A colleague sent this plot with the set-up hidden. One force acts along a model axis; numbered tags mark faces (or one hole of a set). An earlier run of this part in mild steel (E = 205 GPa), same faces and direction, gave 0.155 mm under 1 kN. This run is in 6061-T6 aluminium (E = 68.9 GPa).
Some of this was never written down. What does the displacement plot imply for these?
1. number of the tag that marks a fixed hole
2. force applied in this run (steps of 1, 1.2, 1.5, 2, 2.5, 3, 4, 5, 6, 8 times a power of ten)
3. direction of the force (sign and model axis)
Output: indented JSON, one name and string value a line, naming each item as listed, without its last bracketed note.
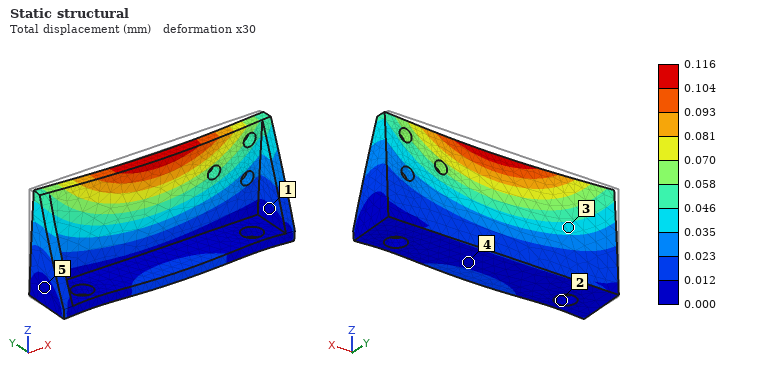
{
  "number of the tag that marks a fixed hole": "2",
  "force applied in this run": "250 N",
  "direction of the force": "-Y"
}
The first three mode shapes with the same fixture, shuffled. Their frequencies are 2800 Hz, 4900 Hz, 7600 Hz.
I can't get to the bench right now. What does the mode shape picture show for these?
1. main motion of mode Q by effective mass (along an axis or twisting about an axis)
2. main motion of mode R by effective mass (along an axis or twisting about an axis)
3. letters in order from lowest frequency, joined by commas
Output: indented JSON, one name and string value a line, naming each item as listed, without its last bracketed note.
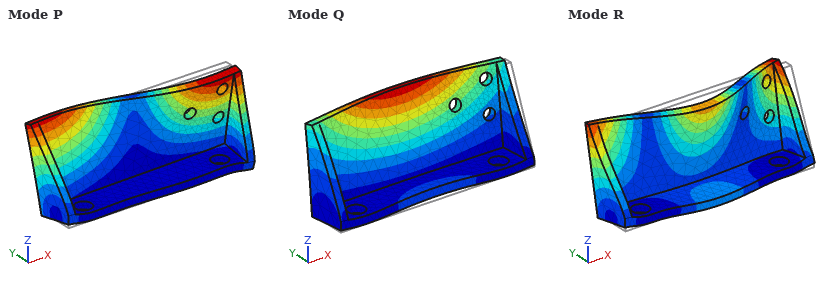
{
  "main motion of mode Q by effective mass": "along Y",
  "main motion of mode R by effective mass": "along Z",
  "letters in order from lowest frequency, joined by commas": "Q, P, R"
}
